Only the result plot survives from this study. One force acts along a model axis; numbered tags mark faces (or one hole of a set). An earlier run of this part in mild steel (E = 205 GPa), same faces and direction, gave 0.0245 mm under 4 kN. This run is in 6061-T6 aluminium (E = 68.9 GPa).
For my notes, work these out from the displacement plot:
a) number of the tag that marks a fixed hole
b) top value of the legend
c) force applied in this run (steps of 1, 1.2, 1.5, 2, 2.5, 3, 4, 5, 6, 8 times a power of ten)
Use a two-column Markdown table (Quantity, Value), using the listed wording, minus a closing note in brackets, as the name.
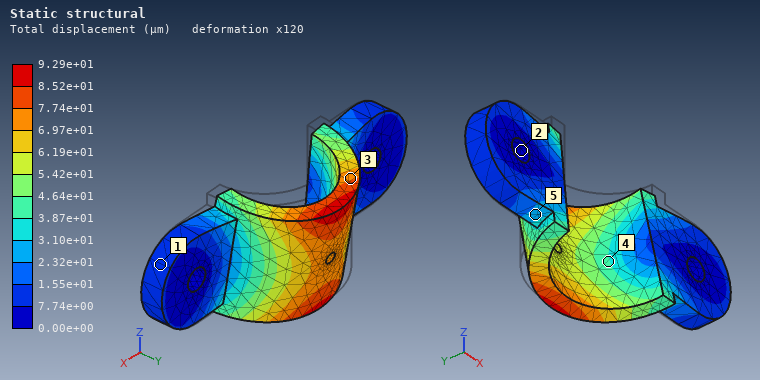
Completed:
| Quantity | Value |
|---|---|
| number of the tag that marks a fixed hole | 2 |
| top value of the legend | 9.29e+01 µm |
| force applied in this run | 5 kN |
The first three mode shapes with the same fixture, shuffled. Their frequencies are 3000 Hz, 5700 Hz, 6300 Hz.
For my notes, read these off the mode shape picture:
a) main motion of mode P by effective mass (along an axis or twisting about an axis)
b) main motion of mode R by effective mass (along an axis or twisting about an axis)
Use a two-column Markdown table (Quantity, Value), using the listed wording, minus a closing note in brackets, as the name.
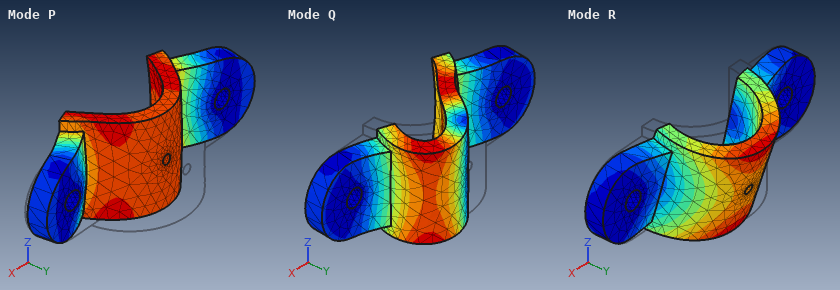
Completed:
| Quantity | Value |
|---|---|
| main motion of mode P by effective mass | along Y |
| main motion of mode R by effective mass | along Z |
